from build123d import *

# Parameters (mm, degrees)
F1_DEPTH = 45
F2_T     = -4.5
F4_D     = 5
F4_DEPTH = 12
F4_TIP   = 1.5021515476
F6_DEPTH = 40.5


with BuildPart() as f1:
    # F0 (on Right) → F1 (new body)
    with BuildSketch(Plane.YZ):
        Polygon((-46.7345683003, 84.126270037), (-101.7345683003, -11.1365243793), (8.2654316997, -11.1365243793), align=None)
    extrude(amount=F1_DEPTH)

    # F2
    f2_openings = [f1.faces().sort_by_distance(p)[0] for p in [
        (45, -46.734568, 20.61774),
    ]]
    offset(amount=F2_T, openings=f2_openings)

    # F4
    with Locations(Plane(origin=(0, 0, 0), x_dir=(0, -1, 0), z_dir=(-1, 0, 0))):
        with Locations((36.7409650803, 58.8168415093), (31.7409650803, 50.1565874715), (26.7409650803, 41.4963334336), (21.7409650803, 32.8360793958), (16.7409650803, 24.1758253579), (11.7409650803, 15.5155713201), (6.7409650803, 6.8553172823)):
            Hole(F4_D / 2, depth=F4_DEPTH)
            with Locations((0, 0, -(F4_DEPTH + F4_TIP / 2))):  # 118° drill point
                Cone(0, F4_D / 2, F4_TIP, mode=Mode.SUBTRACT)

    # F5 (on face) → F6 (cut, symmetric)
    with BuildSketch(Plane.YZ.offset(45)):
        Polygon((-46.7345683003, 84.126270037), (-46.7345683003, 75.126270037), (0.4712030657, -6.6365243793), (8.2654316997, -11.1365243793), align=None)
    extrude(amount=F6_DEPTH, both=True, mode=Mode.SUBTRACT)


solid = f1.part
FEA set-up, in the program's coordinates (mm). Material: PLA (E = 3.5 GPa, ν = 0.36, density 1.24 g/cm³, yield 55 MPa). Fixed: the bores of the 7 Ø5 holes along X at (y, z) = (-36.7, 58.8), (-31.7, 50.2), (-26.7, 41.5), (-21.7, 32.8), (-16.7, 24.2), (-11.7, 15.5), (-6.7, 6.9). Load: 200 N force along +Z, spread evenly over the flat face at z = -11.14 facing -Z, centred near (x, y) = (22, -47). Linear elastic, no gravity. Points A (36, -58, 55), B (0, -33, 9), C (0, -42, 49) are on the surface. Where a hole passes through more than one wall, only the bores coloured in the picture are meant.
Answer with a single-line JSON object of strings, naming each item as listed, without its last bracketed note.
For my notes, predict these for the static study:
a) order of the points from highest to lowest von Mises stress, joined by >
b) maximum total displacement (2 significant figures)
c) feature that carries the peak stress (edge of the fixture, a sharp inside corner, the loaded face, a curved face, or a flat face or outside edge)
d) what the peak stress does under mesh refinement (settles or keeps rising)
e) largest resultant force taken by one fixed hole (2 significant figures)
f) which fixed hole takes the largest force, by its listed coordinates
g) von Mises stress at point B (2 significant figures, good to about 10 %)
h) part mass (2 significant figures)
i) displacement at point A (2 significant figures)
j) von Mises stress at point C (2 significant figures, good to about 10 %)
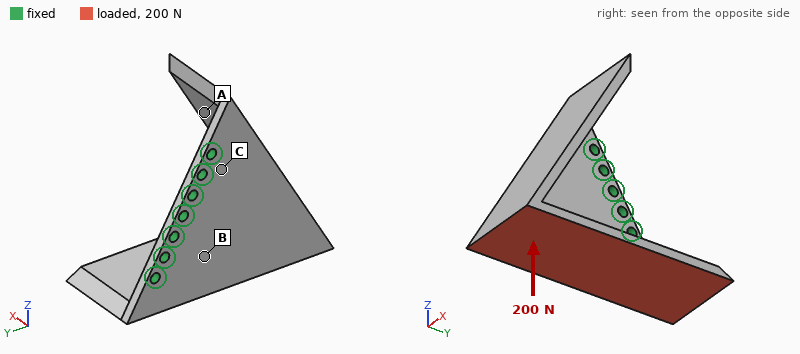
{"order of the points from highest to lowest von Mises stress, joined by >": "B > C > A", "maximum total displacement": "1.6 mm", "feature that carries the peak stress": "edge of the fixture", "what the peak stress does under mesh refinement": "keeps rising", "largest resultant force taken by one fixed hole": "110 N", "which fixed hole takes the largest force, by its listed coordinates": "(-36.7, 58.8)", "von Mises stress at point B": "4.6 MPa", "part mass": "75 g", "displacement at point A": "0.36 mm", "von Mises stress at point C": "2.5 MPa"}
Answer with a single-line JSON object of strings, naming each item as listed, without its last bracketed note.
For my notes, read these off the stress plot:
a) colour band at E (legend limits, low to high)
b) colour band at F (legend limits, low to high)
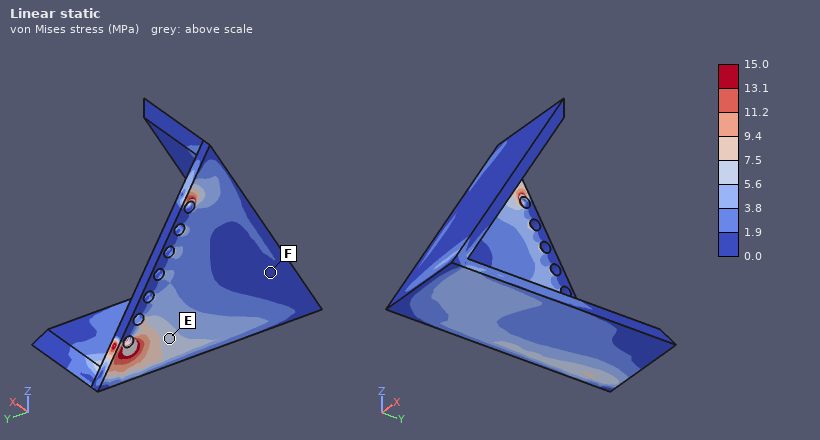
{"colour band at E": "5.6 to 7.5 MPa", "colour band at F": "0.0 to 1.9 MPa"}
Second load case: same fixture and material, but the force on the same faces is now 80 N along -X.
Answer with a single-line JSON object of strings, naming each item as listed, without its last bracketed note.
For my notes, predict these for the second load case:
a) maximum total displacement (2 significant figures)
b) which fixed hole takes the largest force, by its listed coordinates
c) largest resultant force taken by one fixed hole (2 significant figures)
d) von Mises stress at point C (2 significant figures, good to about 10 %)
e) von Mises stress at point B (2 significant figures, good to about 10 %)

{"maximum total displacement": "1.5 mm", "which fixed hole takes the largest force, by its listed coordinates": "(-6.7, 6.9)", "largest resultant force taken by one fixed hole": "40 N", "von Mises stress at point C": "6.3 MPa", "von Mises stress at point B": "3.2 MPa"}
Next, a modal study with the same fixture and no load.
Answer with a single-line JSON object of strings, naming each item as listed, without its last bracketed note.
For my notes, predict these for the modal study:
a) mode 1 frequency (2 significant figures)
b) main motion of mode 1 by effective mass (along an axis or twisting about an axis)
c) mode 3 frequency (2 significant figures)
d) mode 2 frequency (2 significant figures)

{"mode 1 frequency": "180 Hz", "main motion of mode 1 by effective mass": "along X", "mode 3 frequency": "550 Hz", "mode 2 frequency": "440 Hz"}
